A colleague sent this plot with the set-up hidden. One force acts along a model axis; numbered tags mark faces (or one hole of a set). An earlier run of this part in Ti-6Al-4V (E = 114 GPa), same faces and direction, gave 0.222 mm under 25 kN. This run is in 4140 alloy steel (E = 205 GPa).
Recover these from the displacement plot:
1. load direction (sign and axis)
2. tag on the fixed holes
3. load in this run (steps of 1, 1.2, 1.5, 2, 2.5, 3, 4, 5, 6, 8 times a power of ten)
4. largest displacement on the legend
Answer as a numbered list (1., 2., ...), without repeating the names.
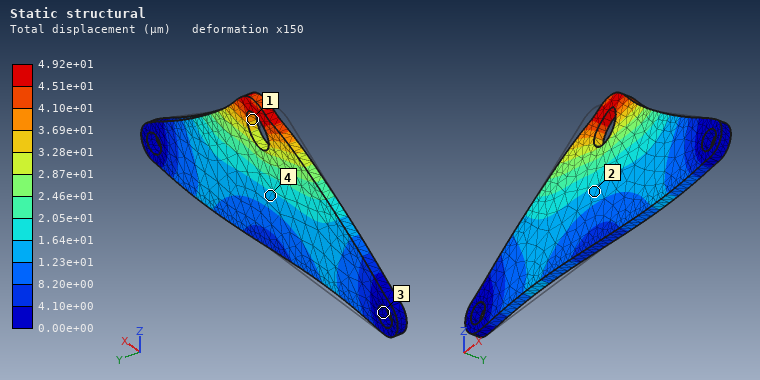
1. +X
2. 3
3. 10 kN
4. 4.92e+01 µm
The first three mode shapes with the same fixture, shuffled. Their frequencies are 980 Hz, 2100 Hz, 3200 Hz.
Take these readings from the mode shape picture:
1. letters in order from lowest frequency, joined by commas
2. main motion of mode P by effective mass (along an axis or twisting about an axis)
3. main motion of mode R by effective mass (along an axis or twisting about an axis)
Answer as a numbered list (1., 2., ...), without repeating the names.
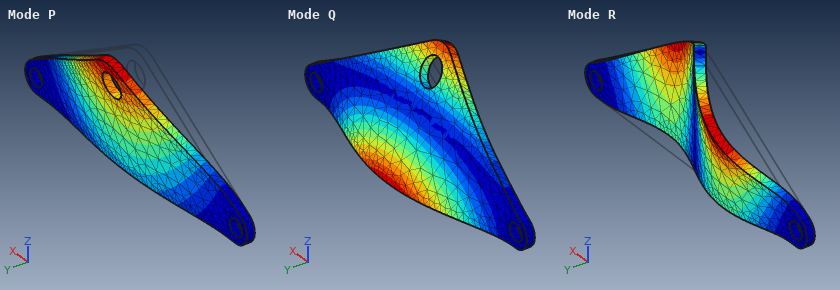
1. P, Q, R
2. along Y
3. twisting about Z
